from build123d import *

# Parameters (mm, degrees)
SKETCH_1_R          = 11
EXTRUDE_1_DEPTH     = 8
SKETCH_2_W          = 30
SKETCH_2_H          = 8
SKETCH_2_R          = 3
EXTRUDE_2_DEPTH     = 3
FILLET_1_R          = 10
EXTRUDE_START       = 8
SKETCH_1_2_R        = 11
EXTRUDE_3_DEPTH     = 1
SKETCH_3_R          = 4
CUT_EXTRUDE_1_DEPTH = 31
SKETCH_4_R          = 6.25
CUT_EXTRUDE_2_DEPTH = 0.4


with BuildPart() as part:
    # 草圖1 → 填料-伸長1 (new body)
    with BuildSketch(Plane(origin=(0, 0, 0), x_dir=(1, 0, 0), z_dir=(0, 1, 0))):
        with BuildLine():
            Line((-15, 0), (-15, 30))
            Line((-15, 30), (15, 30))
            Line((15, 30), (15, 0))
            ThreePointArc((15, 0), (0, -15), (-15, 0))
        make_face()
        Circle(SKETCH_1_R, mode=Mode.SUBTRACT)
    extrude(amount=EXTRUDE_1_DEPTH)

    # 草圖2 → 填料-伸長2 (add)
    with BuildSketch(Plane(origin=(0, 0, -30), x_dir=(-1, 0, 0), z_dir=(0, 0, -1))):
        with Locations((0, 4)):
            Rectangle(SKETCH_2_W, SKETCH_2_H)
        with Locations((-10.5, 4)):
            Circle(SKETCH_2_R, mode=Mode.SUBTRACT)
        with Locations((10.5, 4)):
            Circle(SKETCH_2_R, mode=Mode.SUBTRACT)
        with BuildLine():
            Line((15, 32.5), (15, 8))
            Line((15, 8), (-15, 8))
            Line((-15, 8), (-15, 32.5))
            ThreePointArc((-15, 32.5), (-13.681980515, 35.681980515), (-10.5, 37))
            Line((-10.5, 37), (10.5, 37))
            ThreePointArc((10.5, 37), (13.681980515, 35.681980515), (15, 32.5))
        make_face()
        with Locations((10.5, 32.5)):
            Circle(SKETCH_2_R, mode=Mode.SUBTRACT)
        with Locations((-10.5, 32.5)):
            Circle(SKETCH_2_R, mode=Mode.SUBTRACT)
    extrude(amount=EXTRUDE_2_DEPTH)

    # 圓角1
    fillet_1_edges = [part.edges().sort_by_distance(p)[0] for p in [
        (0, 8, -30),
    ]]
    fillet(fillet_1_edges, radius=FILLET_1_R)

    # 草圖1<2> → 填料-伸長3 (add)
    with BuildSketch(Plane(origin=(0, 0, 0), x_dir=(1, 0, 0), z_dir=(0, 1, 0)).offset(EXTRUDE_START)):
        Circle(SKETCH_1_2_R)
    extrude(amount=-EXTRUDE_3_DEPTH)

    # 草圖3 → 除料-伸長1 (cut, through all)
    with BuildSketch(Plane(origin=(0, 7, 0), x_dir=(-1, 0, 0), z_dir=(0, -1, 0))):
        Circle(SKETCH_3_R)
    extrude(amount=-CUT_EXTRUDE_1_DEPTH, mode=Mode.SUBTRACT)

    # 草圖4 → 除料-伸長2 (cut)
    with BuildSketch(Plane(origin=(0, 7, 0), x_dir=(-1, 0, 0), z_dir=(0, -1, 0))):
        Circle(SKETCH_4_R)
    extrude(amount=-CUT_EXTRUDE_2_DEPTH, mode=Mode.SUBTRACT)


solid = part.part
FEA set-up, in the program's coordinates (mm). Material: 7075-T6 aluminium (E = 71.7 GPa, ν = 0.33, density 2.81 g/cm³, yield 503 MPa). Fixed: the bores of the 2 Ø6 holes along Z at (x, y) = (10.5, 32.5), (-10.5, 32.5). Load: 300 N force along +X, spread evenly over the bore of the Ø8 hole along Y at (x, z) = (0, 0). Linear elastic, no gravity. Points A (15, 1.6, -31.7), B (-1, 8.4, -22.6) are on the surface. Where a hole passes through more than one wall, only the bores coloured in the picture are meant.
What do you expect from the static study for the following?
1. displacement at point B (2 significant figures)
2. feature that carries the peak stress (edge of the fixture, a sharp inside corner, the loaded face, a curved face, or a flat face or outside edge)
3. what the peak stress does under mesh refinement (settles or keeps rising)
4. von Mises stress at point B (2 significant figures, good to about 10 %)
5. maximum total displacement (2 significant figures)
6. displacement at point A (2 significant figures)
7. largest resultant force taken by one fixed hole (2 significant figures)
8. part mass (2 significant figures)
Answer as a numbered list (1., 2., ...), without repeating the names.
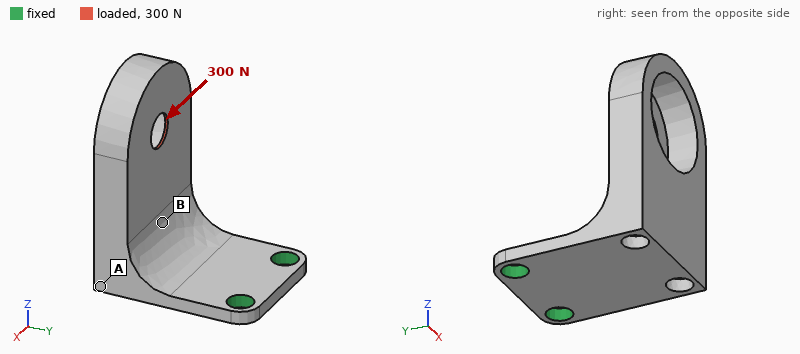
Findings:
1. 0.081 mm
2. edge of the fixture
3. keeps rising
4. 26 MPa
5. 0.42 mm
6. 0.13 mm
7. 540 N
8. 31 g
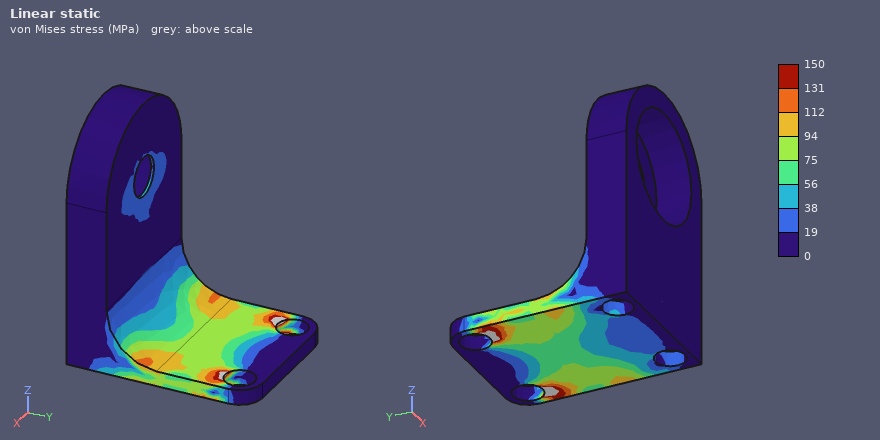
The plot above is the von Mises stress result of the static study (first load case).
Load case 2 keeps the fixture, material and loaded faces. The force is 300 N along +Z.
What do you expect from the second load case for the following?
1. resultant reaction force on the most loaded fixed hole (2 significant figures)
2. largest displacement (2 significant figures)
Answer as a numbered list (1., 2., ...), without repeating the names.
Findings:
1. 150 N
2. 0.76 mm
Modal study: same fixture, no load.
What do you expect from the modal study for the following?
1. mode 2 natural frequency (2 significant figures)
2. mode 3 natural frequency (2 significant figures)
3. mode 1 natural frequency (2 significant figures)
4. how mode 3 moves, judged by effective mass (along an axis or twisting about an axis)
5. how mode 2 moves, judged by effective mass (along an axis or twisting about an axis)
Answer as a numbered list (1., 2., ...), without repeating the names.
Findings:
1. 1400 Hz
2. 3500 Hz
3. 630 Hz
4. along Z
5. along X
